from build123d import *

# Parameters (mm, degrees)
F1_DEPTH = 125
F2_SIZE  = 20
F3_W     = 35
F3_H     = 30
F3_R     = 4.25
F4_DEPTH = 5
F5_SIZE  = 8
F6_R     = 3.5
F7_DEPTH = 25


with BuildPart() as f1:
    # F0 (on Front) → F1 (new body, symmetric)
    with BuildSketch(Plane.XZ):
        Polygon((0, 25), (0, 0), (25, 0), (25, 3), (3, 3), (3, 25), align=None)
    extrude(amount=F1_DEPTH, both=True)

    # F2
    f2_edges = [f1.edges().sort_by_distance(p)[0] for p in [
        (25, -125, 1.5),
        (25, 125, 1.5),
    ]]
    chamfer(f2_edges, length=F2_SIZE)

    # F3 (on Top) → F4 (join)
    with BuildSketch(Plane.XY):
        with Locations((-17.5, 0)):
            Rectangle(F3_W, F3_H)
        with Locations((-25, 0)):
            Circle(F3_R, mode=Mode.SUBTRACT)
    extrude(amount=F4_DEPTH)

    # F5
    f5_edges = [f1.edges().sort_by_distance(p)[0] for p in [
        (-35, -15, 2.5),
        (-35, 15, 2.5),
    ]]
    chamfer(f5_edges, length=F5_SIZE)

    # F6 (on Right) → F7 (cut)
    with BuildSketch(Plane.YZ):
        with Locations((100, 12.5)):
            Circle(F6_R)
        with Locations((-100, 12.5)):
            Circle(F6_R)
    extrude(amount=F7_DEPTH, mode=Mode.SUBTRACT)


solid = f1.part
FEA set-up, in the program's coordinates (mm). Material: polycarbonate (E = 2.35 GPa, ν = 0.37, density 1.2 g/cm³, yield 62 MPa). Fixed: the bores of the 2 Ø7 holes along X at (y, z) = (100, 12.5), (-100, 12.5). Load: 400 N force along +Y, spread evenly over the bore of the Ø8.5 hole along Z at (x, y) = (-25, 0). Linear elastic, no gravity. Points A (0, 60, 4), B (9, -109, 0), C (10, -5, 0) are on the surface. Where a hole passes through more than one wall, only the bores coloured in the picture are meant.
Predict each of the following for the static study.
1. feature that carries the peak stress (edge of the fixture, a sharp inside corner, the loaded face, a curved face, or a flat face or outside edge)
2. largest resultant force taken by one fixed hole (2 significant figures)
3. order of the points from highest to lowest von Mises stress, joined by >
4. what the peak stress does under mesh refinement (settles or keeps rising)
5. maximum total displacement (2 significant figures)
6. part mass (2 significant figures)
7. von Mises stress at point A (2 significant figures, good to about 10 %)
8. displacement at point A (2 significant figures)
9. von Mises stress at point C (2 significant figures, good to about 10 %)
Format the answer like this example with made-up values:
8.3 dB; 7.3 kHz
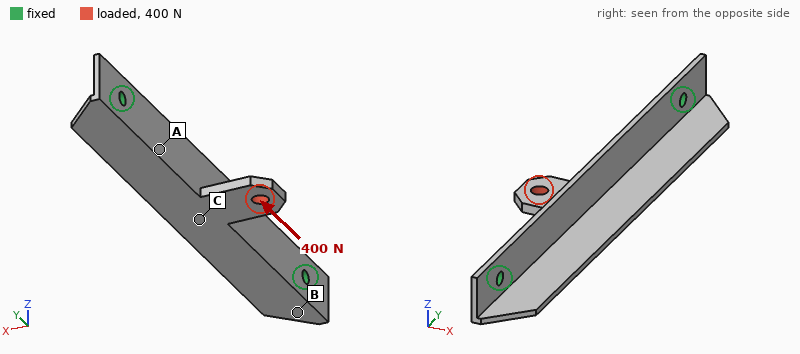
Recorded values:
a sharp inside corner; 210 N; C > A > B; keeps rising; 1.3 mm; 46 g; 5.8 MPa; 0.37 mm; 11 MPa
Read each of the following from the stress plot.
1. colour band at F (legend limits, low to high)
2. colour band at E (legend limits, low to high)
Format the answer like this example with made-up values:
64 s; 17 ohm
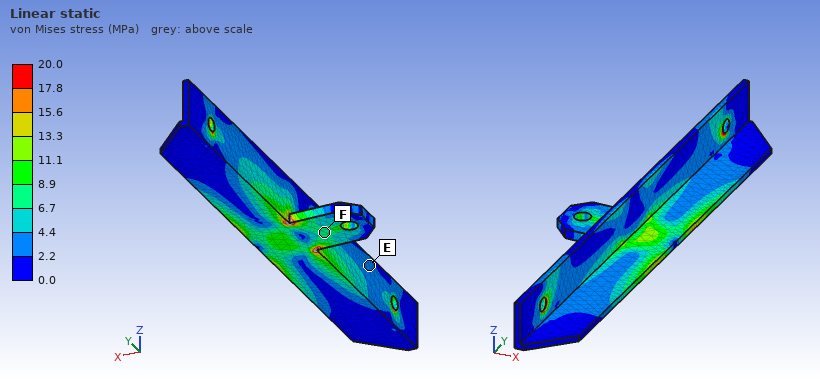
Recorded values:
6.7 to 8.9 MPa; 2.2 to 4.4 MPa
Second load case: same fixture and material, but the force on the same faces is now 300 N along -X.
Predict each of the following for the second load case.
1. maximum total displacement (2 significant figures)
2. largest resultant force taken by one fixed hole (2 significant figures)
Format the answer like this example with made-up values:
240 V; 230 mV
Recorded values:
2.8 mm; 340 N
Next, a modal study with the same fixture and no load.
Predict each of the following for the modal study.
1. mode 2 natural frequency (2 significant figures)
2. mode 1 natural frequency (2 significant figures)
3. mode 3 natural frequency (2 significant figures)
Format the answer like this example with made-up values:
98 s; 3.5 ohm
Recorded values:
340 Hz; 210 Hz; 510 Hz
